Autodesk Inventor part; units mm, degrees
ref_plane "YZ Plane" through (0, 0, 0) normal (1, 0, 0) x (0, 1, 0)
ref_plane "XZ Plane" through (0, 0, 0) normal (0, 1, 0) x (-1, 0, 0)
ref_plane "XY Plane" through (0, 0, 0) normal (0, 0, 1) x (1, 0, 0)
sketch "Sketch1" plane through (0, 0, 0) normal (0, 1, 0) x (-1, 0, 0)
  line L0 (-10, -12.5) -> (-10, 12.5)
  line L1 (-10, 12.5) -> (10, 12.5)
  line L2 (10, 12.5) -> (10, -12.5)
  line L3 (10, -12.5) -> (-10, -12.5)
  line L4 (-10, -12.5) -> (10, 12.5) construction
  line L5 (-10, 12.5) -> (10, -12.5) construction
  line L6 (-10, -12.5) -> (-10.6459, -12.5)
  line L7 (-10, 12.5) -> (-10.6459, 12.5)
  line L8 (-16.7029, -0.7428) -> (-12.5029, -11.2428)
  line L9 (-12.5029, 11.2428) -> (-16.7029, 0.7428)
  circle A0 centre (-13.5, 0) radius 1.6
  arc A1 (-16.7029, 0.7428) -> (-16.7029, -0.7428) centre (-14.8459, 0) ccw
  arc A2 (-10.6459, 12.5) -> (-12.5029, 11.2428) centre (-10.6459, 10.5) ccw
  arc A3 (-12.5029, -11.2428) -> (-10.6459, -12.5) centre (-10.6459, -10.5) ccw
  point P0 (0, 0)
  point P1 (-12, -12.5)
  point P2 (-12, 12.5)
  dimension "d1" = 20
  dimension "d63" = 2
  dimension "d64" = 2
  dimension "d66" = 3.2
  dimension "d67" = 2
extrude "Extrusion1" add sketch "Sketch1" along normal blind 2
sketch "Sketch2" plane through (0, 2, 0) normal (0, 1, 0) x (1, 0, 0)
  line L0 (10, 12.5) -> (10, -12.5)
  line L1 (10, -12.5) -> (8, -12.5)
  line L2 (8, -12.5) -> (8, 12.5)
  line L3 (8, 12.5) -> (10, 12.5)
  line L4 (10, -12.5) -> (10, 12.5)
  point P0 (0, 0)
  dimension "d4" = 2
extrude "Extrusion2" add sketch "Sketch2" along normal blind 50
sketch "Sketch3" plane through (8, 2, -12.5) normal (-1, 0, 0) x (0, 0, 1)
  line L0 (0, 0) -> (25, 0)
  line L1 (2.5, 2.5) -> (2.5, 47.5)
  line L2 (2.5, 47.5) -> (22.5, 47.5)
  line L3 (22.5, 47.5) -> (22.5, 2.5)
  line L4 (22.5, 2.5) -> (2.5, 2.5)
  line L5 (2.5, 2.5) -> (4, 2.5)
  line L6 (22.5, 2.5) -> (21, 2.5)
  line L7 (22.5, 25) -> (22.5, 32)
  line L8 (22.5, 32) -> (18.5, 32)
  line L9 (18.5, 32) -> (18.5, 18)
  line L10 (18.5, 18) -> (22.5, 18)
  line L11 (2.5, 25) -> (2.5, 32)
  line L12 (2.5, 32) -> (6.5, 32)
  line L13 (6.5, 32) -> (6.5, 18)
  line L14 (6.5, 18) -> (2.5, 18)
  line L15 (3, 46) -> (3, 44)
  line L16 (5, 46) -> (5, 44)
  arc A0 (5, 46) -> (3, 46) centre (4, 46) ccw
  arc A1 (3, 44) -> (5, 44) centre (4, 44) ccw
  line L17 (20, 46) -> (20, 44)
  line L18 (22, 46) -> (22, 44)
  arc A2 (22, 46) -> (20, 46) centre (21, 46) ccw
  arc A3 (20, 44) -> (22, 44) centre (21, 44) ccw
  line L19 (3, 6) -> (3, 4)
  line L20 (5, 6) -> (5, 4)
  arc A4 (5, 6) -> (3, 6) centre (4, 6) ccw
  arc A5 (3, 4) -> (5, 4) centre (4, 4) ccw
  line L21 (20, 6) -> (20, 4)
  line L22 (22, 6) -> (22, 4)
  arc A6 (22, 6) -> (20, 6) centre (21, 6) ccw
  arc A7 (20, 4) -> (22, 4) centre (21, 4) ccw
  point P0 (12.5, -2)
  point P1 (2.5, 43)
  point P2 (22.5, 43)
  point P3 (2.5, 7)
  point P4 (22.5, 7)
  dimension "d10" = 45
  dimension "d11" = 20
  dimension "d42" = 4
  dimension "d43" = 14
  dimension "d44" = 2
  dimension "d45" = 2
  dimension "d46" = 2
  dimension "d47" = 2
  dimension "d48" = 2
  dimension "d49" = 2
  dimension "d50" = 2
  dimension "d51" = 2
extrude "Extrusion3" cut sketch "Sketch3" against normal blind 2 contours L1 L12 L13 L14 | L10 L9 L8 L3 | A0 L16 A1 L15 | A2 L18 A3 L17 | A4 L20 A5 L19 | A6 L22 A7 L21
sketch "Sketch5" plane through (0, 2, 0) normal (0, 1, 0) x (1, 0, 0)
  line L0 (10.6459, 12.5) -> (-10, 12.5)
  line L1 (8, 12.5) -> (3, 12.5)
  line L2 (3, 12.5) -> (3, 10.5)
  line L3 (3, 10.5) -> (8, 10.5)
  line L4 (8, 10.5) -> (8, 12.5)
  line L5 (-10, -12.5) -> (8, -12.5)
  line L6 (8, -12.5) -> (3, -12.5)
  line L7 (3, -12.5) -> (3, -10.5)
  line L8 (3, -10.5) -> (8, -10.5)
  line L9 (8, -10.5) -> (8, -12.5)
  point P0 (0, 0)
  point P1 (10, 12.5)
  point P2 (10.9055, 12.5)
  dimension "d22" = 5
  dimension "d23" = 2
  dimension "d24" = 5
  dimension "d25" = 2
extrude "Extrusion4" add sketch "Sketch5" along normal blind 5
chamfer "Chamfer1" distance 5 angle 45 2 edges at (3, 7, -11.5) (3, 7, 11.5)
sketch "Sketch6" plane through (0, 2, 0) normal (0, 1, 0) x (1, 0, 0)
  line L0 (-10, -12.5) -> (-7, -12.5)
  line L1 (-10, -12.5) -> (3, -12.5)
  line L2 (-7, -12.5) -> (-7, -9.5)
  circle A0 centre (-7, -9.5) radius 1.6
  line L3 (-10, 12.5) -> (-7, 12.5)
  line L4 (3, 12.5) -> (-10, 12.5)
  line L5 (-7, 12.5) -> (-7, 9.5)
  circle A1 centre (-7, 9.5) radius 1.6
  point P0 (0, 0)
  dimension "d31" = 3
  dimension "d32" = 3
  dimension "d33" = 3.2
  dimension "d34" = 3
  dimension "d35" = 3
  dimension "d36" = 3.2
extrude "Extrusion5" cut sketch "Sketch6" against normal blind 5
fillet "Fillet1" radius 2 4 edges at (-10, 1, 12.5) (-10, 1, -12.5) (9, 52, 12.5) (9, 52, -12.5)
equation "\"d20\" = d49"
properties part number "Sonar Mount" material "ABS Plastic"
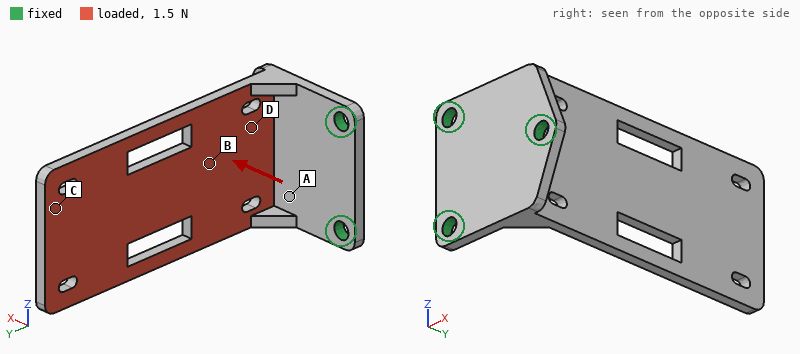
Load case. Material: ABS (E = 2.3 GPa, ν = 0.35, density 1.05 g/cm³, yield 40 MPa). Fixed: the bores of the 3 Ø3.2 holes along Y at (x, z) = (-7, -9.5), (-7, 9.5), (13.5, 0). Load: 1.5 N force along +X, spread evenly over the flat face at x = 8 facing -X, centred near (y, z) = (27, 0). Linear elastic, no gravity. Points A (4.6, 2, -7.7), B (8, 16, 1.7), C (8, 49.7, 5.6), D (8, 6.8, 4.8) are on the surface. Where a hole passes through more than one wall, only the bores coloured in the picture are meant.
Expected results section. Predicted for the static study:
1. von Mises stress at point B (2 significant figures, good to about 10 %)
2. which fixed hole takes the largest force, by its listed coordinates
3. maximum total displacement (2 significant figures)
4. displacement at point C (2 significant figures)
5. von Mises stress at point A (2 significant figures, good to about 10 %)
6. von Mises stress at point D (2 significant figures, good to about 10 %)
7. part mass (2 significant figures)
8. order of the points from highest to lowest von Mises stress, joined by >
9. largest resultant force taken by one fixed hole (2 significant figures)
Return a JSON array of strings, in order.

["1.2 MPa", "(13.5, 0)", "0.71 mm", "0.67 mm", "0.60 MPa", "1.7 MPa", "3.6 g", "D > B > A > C", "2.6 N"]
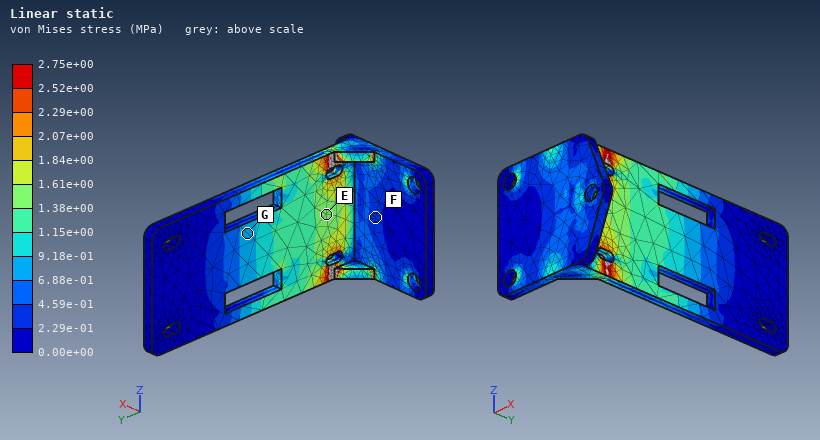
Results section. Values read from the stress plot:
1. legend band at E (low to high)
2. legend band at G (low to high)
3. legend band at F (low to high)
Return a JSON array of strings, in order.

["1.38e+00 to 1.61e+00 MPa", "6.88e-01 to 9.18e-01 MPa", "2.29e-01 to 4.59e-01 MPa"]
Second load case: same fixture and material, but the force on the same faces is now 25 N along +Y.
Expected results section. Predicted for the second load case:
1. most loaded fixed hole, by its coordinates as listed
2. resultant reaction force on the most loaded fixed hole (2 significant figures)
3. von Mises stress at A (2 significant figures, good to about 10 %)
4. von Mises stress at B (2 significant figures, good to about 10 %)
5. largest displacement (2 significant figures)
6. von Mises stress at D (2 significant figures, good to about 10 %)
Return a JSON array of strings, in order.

["(13.5, 0)", "20 N", "1.2 MPa", "1.7 MPa", "0.68 mm", "1.7 MPa"]
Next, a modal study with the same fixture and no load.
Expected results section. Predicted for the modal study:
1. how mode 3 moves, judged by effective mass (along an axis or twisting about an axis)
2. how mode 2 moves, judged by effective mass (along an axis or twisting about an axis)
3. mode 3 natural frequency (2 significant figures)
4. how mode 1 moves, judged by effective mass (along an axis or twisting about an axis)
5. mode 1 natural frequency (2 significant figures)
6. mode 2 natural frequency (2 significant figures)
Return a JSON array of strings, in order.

["twisting about Y", "along Z", "790 Hz", "along X", "190 Hz", "540 Hz"]
